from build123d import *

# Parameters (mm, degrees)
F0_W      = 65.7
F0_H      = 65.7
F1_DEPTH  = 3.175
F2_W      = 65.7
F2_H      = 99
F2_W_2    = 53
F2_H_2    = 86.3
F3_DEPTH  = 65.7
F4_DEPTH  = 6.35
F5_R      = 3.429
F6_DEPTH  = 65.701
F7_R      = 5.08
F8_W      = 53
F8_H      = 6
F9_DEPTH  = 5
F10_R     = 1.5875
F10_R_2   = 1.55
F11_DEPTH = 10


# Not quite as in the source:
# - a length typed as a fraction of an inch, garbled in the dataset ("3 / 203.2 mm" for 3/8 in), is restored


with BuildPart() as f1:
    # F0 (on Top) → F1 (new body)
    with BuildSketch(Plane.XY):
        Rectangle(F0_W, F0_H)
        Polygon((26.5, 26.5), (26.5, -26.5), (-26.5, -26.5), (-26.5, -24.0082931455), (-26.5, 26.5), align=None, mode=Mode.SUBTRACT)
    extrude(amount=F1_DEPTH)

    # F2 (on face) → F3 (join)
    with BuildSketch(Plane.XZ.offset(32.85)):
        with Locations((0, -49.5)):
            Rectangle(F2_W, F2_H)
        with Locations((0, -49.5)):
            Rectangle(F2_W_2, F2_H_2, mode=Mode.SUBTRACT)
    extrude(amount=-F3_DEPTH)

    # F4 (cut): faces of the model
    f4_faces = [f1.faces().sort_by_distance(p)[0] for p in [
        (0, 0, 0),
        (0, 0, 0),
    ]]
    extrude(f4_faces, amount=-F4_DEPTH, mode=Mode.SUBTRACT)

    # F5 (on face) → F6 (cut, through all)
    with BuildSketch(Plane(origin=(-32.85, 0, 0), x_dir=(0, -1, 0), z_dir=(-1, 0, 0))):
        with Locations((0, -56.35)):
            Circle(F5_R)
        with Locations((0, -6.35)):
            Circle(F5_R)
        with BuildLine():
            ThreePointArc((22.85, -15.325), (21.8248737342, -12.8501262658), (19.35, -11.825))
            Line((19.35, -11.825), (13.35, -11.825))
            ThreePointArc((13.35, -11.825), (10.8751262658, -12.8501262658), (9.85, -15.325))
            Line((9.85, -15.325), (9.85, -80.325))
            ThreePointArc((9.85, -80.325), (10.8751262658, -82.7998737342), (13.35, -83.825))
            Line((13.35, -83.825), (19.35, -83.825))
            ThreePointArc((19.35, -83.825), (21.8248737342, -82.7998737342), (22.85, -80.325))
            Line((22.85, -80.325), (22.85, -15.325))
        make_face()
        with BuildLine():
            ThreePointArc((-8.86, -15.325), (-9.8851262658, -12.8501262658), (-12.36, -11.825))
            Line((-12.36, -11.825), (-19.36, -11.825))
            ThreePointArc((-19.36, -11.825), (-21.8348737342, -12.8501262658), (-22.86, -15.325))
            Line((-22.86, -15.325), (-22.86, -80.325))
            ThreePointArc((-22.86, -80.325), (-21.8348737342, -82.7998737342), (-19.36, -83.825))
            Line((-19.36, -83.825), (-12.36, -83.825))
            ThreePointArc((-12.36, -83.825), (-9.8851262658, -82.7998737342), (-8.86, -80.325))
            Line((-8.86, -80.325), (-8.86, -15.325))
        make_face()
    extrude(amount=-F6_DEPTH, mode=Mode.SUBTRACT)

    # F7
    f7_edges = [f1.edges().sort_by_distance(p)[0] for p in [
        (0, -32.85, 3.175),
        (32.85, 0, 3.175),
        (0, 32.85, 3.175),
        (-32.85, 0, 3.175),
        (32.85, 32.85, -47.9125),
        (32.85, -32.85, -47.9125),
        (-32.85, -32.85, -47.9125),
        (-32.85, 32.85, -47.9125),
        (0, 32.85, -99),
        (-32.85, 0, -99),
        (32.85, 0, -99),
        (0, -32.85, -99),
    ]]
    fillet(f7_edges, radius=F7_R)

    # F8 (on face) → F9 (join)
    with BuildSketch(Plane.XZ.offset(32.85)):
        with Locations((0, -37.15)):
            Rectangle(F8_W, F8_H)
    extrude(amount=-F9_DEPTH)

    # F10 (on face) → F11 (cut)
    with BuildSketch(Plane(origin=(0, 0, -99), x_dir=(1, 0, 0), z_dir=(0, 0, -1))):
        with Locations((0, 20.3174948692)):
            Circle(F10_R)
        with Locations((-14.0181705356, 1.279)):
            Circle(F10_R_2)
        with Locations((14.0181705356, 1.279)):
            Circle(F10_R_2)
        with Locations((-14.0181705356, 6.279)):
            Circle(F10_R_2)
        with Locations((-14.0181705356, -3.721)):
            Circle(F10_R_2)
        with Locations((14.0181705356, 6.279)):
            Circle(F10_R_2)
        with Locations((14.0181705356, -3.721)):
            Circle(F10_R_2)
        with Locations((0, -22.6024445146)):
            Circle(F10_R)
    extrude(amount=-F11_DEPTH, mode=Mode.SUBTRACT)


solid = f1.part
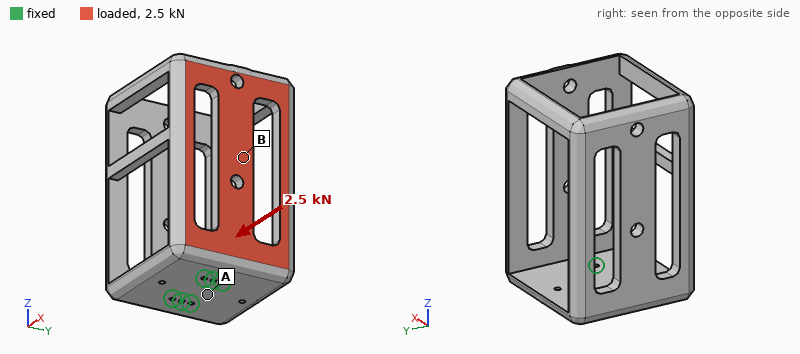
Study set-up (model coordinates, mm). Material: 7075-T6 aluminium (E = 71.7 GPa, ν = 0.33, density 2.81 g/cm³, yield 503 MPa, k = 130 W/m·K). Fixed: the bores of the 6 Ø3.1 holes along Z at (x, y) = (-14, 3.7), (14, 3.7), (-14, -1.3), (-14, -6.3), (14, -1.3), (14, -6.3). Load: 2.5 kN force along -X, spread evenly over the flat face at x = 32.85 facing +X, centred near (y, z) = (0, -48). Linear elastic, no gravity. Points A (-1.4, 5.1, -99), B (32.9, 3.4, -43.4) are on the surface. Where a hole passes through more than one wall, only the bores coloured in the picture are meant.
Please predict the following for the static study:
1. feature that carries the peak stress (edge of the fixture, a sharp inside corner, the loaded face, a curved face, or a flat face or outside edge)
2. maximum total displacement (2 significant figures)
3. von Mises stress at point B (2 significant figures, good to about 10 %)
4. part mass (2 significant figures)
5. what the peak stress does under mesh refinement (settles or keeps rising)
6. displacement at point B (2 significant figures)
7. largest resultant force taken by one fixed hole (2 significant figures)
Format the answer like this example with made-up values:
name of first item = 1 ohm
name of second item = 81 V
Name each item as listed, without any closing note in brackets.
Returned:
feature that carries the peak stress = edge of the fixture
maximum total displacement = 1.3 mm
von Mises stress at point B = 49 MPa
part mass = 240 g
what the peak stress does under mesh refinement = keeps rising
displacement at point B = 0.83 mm
largest resultant force taken by one fixed hole = 1.2 kN
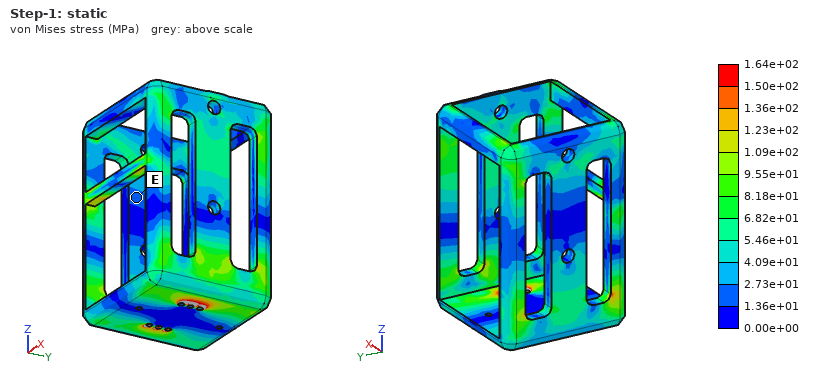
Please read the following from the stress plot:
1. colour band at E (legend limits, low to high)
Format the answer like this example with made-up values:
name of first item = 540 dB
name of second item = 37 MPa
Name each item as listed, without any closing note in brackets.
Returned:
colour band at E = 1.36e+01 to 2.73e+01 MPa
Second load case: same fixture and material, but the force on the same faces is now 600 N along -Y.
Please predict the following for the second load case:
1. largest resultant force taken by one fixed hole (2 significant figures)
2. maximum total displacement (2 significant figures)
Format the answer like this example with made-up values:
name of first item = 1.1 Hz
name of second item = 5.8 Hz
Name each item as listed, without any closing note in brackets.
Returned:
largest resultant force taken by one fixed hole = 1.0 kN
maximum total displacement = 0.22 mm
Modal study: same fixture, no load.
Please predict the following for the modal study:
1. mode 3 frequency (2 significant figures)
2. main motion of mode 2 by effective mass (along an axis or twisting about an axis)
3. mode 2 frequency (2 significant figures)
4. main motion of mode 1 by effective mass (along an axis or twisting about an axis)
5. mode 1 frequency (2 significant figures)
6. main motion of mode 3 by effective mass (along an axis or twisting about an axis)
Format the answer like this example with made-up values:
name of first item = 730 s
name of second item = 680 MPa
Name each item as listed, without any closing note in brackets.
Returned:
mode 3 frequency = 1200 Hz
main motion of mode 2 by effective mass = along Y
mode 2 frequency = 790 Hz
main motion of mode 1 by effective mass = along X
mode 1 frequency = 570 Hz
main motion of mode 3 by effective mass = twisting about Z
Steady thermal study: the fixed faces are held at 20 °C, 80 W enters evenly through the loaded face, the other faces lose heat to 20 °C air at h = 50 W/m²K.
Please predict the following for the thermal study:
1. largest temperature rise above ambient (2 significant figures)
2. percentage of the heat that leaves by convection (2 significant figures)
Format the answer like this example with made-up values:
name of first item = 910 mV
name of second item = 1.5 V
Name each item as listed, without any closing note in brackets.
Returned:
largest temperature rise above ambient = 67 K
percentage of the heat that leaves by convection = 43 %
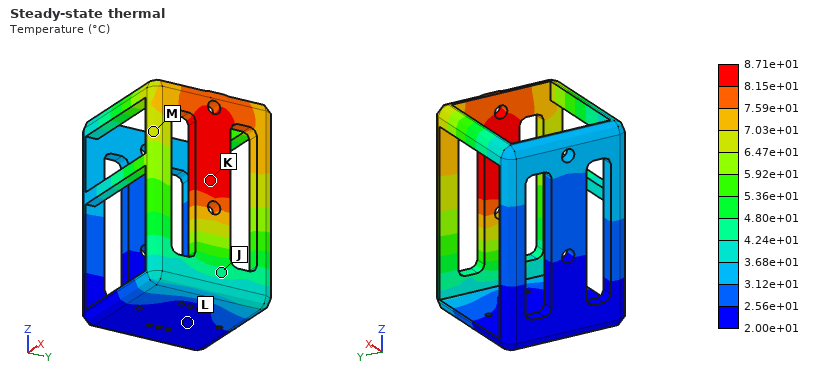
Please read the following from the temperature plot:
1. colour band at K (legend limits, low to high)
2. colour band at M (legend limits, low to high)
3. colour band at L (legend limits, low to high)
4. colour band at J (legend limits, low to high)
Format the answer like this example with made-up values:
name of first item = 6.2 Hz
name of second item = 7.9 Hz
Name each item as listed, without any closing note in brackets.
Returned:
colour band at K = 8.15e+01 to 8.71e+01 °C
colour band at M = 6.47e+01 to 7.03e+01 °C
colour band at L = 2.00e+01 to 2.56e+01 °C
colour band at J = 4.24e+01 to 4.80e+01 °C
